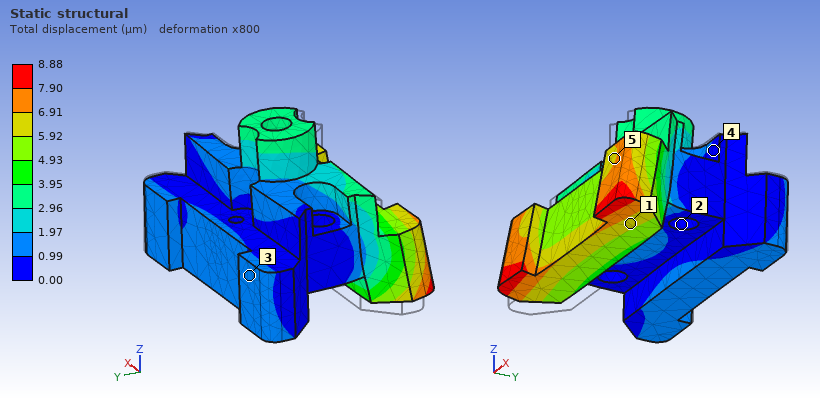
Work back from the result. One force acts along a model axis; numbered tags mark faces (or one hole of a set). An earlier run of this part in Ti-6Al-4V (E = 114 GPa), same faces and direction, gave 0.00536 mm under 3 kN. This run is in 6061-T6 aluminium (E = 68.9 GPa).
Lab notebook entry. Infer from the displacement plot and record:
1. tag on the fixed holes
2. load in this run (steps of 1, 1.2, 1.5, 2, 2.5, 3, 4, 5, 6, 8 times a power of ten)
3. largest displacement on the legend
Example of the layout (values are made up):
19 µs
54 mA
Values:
2
3 kN
8.88 µm
